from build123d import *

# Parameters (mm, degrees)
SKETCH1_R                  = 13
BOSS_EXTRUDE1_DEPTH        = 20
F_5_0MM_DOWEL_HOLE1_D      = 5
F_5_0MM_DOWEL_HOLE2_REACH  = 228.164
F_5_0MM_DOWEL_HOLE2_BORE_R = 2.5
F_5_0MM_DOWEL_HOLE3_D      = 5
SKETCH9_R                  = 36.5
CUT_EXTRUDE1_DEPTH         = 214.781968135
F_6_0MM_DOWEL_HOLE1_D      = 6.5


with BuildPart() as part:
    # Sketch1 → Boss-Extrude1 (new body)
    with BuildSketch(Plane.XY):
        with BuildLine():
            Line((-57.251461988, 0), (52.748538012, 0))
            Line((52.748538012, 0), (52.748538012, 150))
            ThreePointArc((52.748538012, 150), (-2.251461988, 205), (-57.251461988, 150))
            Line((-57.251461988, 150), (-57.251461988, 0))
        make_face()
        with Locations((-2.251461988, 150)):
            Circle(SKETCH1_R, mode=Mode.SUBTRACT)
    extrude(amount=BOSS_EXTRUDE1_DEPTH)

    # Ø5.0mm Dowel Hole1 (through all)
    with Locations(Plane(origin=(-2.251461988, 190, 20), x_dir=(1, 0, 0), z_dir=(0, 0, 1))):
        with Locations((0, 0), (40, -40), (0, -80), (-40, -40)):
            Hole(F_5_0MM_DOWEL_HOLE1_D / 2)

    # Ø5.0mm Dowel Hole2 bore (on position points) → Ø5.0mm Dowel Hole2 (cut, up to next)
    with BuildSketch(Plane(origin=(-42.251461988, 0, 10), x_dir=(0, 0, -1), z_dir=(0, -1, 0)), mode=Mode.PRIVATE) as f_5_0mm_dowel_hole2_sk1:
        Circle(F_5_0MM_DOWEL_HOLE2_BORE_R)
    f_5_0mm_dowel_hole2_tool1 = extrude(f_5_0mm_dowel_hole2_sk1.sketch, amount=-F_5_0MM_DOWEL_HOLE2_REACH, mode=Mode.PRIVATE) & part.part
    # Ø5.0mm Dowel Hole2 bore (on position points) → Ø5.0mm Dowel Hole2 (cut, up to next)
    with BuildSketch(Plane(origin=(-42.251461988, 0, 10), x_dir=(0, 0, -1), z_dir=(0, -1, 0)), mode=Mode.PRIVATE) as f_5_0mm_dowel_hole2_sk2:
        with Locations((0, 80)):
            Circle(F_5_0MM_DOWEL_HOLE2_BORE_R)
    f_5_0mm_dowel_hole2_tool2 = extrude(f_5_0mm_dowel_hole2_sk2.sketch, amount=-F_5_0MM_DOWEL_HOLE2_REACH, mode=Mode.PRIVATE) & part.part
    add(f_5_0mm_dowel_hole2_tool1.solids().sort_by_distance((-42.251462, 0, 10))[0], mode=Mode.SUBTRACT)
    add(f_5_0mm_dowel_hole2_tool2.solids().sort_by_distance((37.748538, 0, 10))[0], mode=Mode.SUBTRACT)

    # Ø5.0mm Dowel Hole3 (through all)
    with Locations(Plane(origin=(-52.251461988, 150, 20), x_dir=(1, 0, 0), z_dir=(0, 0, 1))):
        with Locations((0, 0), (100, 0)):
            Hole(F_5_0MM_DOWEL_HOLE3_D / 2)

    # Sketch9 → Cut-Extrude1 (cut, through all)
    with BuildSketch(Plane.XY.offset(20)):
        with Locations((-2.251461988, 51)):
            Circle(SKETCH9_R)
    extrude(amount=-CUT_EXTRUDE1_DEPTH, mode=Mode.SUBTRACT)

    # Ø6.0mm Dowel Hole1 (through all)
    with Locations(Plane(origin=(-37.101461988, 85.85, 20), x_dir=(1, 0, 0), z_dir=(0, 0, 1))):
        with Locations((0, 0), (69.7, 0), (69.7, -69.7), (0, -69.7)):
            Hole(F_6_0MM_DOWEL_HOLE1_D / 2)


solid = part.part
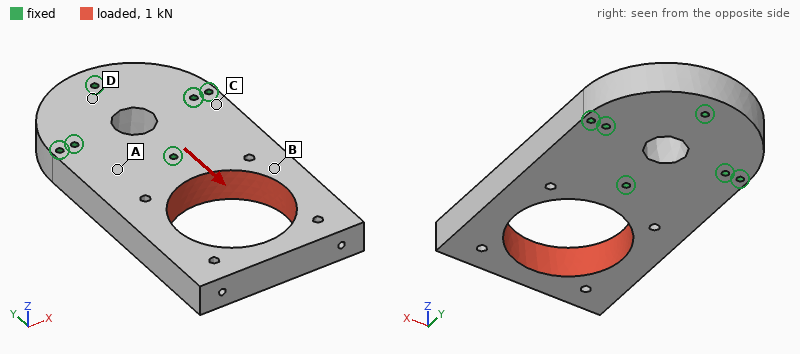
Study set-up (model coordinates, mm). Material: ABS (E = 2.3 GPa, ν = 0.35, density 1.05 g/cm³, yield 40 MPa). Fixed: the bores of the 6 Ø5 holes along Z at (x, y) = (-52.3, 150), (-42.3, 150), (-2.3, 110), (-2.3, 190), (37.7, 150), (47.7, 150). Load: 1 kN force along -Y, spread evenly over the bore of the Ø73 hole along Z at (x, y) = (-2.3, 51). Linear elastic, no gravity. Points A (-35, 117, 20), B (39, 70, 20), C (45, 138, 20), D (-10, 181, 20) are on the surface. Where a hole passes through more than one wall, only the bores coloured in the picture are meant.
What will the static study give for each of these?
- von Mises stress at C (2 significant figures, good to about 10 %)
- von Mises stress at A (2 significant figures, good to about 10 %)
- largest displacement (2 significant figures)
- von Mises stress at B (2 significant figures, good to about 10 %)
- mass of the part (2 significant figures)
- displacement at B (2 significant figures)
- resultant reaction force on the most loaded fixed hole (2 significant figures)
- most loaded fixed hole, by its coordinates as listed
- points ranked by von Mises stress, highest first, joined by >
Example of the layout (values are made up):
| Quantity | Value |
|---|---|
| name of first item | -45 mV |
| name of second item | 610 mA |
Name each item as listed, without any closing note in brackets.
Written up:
| Quantity | Value |
|---|---|
| von Mises stress at C | 0.77 MPa |
| von Mises stress at A | 0.46 MPa |
| largest displacement | 98 µm |
| von Mises stress at B | 1.1 MPa |
| mass of the part | 340 g |
| displacement at B | 35 µm |
| resultant reaction force on the most loaded fixed hole | 240 N |
| most loaded fixed hole, by its coordinates as listed | (-2.3, 110) |
| points ranked by von Mises stress, highest first, joined by > | B > C > A > D |
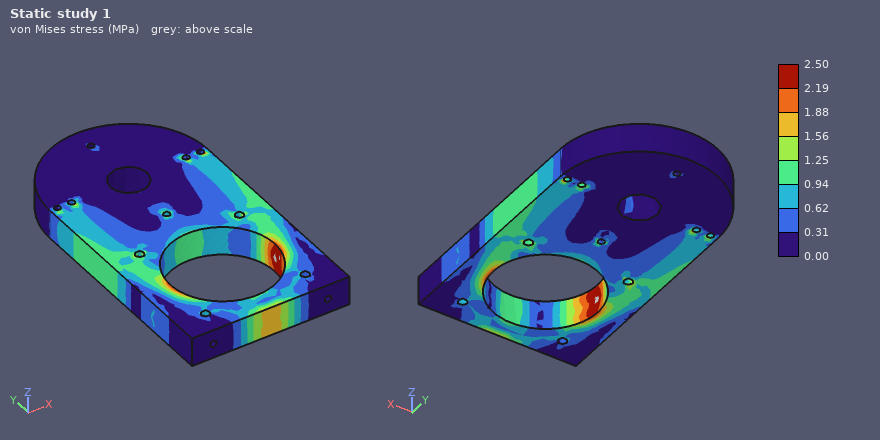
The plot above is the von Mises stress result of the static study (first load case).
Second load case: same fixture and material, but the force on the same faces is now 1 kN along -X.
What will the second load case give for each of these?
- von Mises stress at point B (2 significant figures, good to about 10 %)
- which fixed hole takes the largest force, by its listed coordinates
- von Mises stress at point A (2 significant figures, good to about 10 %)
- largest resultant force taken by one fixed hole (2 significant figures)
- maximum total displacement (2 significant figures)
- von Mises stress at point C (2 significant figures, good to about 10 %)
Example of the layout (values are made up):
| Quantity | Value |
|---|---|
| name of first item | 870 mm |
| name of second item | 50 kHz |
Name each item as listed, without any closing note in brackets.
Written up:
| Quantity | Value |
|---|---|
| von Mises stress at point B | 1.6 MPa |
| which fixed hole takes the largest force, by its listed coordinates | (-2.3, 110) |
| von Mises stress at point A | 0.58 MPa |
| largest resultant force taken by one fixed hole | 1.1 kN |
| maximum total displacement | 0.41 mm |
| von Mises stress at point C | 1.5 MPa |
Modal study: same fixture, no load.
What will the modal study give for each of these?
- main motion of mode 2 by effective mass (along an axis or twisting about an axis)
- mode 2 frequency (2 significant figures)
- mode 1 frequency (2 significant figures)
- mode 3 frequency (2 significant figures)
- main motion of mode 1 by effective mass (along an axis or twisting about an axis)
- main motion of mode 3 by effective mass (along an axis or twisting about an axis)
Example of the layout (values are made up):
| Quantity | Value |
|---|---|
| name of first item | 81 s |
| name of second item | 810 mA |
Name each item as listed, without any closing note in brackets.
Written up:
| Quantity | Value |
|---|---|
| main motion of mode 2 by effective mass | twisting about Y |
| mode 2 frequency | 530 Hz |
| mode 1 frequency | 290 Hz |
| mode 3 frequency | 740 Hz |
| main motion of mode 1 by effective mass | along Z |
| main motion of mode 3 by effective mass | along X |
